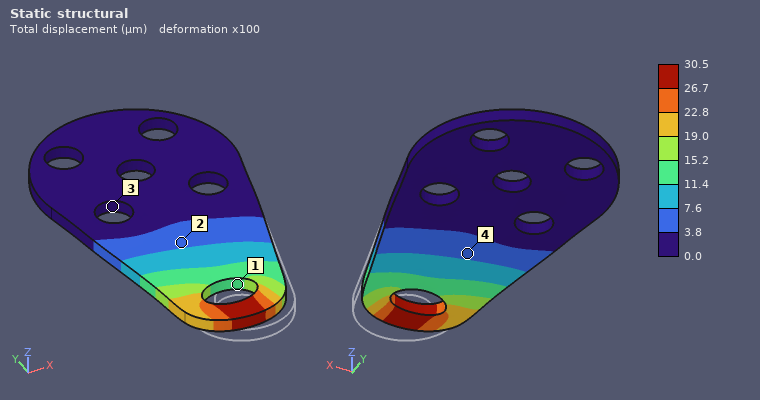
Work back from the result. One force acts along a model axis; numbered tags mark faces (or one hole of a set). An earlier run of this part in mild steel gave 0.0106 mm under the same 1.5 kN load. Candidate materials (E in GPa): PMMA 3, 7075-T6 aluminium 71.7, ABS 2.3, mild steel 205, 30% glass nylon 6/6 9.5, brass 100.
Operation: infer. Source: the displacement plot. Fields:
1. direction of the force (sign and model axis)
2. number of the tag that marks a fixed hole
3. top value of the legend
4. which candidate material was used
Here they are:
+Y
3
30.5 µm
7075-T6 aluminium
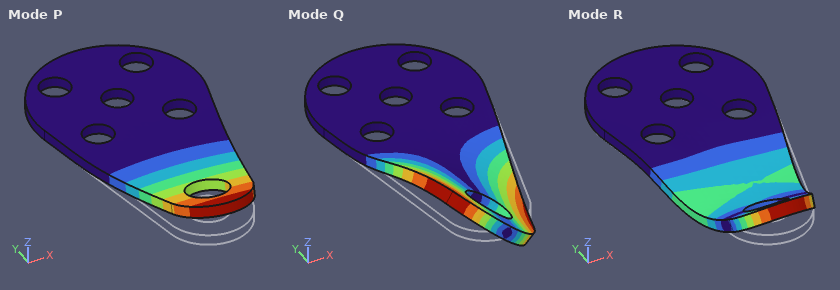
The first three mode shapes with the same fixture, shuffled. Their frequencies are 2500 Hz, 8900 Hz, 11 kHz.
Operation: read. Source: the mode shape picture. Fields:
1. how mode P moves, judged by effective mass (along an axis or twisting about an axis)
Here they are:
along Z
